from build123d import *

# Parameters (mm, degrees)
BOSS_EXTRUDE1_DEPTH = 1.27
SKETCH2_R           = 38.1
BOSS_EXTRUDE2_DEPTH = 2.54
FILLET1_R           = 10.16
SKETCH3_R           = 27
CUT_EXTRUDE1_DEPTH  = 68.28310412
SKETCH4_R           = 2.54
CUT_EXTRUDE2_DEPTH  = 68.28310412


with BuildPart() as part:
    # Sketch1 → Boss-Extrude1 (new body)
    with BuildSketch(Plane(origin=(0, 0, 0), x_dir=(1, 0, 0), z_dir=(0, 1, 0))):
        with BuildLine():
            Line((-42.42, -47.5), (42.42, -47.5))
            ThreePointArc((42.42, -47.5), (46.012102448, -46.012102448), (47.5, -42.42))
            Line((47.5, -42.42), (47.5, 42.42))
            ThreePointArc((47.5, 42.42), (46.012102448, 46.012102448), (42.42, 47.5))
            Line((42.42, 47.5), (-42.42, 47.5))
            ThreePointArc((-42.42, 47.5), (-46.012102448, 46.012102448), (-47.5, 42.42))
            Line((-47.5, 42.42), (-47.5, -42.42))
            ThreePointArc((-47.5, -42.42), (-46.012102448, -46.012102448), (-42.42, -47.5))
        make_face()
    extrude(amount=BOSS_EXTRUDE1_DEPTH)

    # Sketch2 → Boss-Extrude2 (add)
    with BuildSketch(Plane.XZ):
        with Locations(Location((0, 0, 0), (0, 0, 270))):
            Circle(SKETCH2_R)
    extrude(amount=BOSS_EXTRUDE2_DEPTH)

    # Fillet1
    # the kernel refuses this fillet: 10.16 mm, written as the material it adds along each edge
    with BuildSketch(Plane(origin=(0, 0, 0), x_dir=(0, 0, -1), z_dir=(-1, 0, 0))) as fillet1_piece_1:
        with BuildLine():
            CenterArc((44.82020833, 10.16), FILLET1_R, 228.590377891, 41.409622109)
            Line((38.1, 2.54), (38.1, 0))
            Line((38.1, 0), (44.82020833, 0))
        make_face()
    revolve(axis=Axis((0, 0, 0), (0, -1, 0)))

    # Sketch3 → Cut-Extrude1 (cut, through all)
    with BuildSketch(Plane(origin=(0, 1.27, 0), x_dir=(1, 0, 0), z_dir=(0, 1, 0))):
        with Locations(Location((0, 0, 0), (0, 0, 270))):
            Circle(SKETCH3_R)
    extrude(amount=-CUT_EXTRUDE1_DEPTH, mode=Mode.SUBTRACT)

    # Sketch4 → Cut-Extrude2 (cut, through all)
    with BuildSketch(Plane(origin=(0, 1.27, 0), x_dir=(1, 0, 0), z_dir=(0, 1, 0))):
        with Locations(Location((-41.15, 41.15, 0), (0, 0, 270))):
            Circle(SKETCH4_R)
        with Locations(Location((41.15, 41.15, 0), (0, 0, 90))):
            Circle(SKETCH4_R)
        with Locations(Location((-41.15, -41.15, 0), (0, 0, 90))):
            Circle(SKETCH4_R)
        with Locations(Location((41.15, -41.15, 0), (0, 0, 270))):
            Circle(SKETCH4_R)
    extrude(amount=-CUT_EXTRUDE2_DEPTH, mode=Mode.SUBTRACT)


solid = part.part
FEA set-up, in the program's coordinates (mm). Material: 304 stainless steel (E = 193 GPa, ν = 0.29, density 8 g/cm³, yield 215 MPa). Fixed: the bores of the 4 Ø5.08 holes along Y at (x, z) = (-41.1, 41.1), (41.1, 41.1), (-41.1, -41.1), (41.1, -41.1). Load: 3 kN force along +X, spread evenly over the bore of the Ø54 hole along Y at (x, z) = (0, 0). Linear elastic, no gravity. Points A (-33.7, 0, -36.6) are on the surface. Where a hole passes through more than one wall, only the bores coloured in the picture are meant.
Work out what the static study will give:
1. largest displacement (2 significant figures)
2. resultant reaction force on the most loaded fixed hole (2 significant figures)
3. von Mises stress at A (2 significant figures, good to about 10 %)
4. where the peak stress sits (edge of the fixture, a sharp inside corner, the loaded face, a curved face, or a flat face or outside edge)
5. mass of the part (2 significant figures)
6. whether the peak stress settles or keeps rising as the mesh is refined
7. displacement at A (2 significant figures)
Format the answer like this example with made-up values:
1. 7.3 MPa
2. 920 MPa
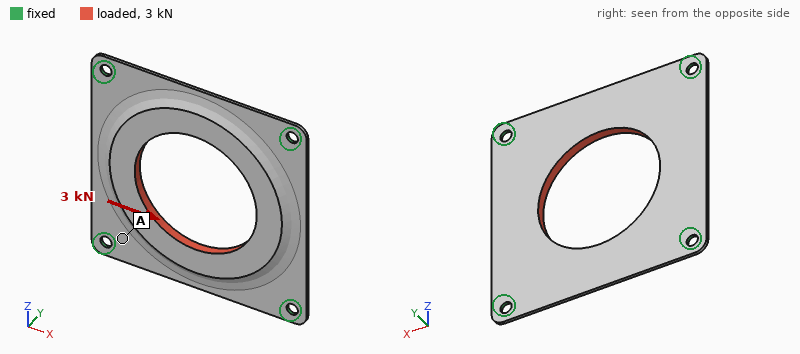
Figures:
1. 8.8 µm
2. 800 N
3. 45 MPa
4. edge of the fixture
5. 120 g
6. keeps rising
7. 4.2 µm
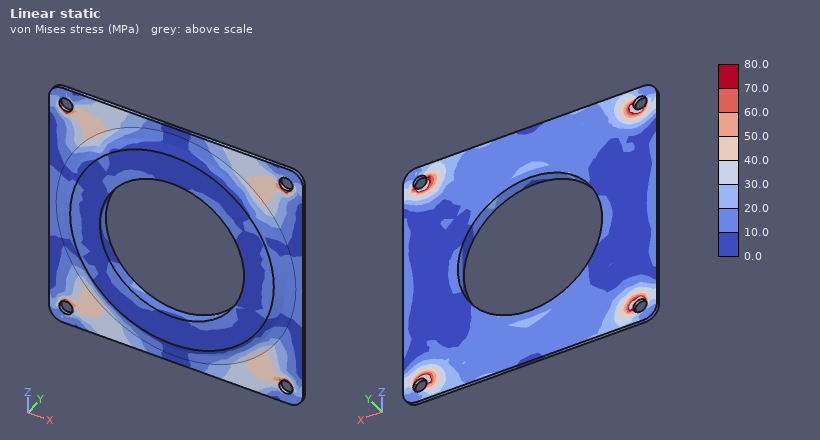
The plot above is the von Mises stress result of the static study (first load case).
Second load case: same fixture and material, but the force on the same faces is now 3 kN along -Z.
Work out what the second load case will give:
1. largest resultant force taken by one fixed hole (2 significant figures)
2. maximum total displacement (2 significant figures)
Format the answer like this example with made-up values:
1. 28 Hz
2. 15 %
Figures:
1. 800 N
2. 8.8 µm
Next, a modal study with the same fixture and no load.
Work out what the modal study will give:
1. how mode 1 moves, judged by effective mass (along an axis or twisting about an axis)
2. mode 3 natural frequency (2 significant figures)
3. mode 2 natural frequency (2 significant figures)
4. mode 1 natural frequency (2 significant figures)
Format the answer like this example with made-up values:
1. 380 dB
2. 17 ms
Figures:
1. along Y
2. 1600 Hz
3. 1600 Hz
4. 1200 Hz
